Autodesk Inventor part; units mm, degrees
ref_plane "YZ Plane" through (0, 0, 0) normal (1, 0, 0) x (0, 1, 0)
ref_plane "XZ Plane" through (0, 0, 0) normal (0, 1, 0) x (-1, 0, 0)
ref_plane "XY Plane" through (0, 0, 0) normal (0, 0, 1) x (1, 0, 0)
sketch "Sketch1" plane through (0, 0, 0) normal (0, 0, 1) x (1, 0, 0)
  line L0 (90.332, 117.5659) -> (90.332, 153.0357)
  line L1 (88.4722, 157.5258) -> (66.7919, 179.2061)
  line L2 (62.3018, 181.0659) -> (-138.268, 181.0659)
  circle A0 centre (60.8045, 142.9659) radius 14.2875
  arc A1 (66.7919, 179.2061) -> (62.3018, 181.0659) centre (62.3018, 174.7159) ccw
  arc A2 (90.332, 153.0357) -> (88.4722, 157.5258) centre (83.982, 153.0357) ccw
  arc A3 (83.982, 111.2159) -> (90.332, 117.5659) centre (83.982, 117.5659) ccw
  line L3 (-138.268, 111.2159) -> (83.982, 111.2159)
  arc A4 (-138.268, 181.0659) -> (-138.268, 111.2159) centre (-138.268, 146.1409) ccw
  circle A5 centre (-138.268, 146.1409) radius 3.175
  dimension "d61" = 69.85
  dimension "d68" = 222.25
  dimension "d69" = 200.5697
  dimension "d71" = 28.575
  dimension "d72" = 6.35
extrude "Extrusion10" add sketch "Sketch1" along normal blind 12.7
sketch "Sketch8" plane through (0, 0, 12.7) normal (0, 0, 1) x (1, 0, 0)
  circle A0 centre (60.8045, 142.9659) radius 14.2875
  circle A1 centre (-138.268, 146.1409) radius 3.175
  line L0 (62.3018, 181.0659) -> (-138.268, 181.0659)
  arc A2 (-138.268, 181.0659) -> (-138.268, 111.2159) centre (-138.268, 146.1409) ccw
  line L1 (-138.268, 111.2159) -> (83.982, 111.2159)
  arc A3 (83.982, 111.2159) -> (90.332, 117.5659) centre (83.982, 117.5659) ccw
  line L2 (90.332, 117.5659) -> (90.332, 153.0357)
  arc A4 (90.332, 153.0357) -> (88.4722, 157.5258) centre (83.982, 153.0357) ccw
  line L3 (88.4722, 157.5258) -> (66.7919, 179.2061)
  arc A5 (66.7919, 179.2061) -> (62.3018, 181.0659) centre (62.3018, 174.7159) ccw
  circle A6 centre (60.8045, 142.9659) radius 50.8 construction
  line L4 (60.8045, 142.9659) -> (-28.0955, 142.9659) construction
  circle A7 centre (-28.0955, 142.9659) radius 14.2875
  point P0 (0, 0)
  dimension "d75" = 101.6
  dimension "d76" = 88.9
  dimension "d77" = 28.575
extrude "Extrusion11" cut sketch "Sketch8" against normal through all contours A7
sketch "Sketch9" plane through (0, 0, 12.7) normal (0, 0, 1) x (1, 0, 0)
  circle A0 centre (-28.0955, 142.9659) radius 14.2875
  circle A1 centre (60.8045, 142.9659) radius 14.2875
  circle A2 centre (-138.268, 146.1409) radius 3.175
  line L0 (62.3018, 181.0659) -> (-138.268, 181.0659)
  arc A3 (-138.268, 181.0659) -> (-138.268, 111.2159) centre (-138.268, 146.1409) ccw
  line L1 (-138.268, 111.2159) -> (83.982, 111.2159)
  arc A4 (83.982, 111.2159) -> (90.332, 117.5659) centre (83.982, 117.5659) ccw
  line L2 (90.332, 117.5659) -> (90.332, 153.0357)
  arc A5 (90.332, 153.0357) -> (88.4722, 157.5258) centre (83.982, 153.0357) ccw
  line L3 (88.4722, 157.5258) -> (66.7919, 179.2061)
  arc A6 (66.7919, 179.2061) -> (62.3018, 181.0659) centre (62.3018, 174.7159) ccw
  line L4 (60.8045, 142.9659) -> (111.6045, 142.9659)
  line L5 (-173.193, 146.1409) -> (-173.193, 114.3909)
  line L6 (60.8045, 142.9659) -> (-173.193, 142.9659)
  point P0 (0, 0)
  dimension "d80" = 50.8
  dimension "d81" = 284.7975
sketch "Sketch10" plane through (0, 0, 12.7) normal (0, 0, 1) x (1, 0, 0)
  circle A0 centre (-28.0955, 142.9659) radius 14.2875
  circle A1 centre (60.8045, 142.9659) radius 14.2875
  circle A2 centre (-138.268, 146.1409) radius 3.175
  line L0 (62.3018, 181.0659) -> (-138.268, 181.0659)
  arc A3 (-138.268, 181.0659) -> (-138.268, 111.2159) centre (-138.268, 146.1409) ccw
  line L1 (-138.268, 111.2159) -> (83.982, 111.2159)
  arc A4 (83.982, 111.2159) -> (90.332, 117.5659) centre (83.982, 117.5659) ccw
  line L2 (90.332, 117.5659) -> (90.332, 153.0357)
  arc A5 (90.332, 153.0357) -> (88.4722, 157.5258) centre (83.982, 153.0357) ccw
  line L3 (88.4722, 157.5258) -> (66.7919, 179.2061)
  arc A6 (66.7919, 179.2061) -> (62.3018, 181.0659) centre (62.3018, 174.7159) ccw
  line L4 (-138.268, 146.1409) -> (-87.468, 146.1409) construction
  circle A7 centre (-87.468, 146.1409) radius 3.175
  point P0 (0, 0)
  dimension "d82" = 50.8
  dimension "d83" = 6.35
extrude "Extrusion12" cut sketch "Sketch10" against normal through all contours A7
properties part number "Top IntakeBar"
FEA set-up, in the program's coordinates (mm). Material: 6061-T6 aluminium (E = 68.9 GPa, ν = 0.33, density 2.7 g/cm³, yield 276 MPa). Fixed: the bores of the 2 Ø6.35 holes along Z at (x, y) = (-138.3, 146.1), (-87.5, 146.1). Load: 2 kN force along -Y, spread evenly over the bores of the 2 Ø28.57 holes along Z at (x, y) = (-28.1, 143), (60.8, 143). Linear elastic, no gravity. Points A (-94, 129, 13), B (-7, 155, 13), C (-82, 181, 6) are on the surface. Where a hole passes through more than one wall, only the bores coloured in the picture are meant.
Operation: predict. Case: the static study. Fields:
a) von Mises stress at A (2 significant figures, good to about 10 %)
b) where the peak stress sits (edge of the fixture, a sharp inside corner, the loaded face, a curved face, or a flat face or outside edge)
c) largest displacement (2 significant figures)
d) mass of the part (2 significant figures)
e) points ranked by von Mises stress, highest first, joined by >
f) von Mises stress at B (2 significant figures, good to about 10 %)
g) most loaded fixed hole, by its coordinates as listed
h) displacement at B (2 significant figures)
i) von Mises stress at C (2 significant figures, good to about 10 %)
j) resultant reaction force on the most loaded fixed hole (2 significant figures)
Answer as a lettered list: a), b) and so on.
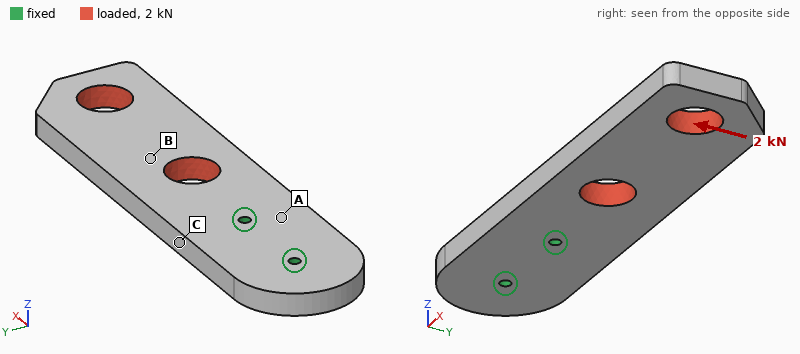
a) 12 MPa
b) edge of the fixture
c) 0.16 mm
d) 560 g
e) C > A > B
f) 4.7 MPa
g) (-87.5, 146.1)
h) 0.065 mm
i) 21 MPa
j) 5.7 kN
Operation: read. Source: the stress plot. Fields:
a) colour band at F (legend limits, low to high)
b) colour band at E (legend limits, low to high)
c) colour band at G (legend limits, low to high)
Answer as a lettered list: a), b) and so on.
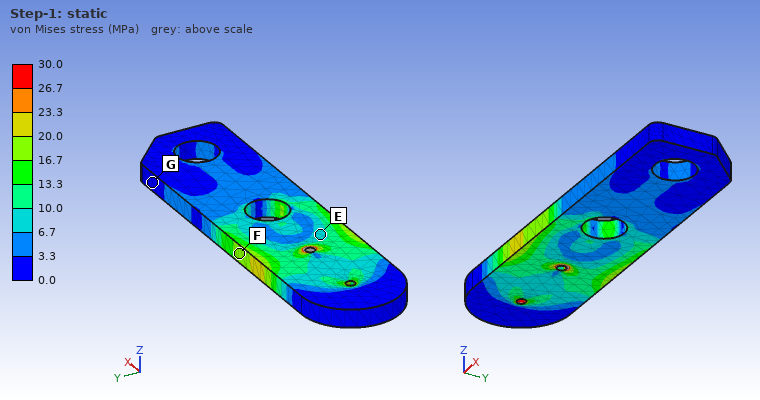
a) 16.7 to 20.0 MPa
b) 6.7 to 10.0 MPa
c) 0.0 to 3.3 MPa
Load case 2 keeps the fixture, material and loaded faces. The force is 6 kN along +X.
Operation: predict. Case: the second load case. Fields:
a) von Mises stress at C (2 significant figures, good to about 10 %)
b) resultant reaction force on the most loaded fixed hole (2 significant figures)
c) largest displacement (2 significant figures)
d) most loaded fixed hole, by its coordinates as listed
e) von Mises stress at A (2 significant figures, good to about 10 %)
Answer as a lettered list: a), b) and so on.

a) 2.8 MPa
b) 4.3 kN
c) 26 µm
d) (-87.5, 146.1)
e) 5.6 MPa
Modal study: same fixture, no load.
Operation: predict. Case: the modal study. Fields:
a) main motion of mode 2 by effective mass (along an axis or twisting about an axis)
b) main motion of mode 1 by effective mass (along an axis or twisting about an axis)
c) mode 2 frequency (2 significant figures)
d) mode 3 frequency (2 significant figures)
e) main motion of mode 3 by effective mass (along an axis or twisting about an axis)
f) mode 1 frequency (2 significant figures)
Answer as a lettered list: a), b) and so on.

a) along Y
b) along Z
c) 1300 Hz
d) 1400 Hz
e) twisting about X
f) 330 Hz
